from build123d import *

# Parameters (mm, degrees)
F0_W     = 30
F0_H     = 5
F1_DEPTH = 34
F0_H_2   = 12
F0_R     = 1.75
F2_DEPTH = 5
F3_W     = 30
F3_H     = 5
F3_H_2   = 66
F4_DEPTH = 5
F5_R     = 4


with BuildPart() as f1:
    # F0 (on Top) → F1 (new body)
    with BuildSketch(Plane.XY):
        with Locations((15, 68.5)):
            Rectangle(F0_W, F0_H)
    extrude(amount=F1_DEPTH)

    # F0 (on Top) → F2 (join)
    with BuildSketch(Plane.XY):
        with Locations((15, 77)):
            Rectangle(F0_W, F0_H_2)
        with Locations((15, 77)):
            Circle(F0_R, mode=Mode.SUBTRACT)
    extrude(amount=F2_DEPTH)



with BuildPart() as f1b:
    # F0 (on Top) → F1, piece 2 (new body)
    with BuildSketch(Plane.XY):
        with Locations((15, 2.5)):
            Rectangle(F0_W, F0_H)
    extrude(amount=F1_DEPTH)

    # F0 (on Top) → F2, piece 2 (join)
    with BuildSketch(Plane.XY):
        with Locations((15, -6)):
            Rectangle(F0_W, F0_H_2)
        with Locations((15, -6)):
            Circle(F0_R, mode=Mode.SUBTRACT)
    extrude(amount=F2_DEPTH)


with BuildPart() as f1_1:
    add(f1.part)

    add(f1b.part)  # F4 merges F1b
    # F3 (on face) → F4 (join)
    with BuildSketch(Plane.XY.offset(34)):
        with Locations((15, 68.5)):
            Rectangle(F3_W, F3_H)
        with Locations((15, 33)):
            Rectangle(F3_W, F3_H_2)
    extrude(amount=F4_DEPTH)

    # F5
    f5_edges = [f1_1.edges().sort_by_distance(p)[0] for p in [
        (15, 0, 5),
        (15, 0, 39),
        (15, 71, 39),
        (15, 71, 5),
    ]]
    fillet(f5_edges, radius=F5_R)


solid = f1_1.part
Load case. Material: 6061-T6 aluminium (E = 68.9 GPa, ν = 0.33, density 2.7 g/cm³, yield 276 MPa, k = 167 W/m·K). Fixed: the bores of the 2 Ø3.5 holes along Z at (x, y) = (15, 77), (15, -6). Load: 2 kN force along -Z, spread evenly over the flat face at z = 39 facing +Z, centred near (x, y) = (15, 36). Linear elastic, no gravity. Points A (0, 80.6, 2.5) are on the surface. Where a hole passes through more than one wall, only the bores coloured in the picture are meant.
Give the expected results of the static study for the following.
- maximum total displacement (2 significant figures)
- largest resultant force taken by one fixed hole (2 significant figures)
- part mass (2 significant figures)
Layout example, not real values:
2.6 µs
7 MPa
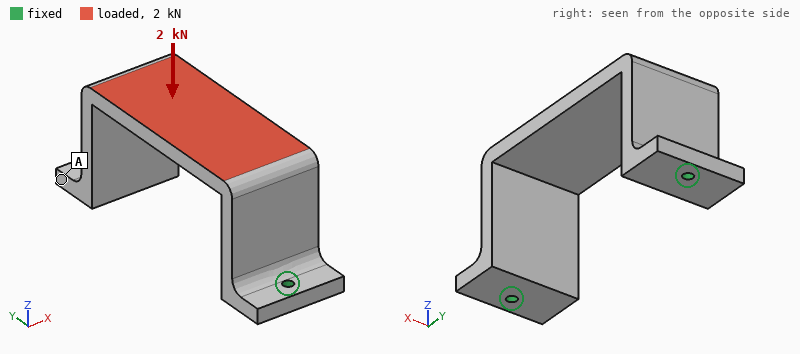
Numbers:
0.13 mm
1.1 kN
66 g
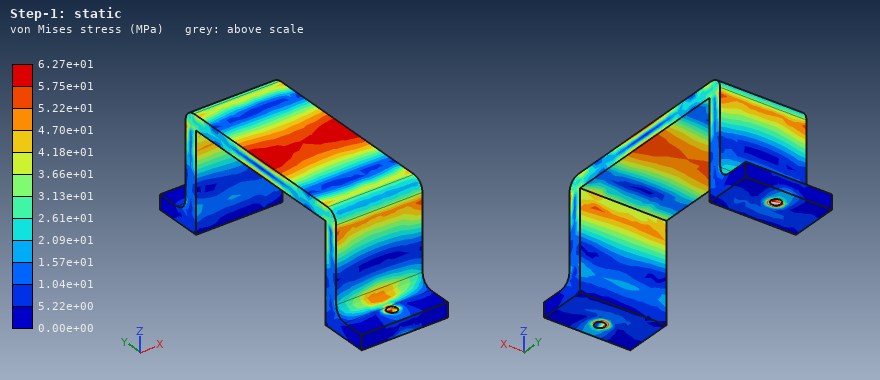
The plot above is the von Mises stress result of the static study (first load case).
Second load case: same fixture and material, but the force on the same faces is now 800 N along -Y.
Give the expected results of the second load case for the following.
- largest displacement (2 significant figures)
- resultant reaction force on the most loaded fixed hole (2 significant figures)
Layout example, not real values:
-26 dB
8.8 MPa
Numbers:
0.13 mm
460 N
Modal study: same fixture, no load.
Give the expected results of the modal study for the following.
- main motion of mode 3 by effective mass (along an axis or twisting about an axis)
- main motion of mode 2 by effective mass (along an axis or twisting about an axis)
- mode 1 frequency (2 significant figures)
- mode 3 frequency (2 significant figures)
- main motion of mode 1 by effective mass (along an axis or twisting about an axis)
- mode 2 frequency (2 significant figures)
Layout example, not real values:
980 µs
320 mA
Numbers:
twisting about Z
along Y
1800 Hz
3100 Hz
along X
2100 Hz
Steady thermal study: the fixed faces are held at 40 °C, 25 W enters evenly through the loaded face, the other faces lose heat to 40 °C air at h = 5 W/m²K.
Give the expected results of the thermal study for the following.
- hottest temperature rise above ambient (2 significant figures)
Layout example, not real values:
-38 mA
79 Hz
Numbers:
29 K
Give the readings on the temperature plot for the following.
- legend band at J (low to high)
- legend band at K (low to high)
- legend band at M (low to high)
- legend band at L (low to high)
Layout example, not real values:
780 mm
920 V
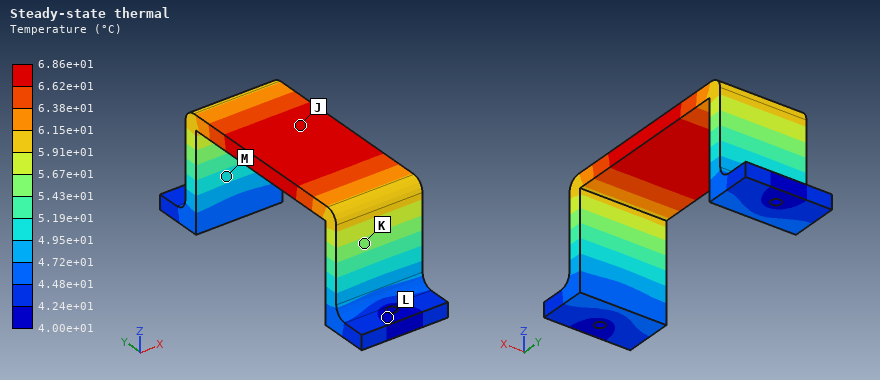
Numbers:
6.62e+01 to 6.86e+01 °C
5.43e+01 to 5.67e+01 °C
4.95e+01 to 5.19e+01 °C
4.00e+01 to 4.24e+01 °C
